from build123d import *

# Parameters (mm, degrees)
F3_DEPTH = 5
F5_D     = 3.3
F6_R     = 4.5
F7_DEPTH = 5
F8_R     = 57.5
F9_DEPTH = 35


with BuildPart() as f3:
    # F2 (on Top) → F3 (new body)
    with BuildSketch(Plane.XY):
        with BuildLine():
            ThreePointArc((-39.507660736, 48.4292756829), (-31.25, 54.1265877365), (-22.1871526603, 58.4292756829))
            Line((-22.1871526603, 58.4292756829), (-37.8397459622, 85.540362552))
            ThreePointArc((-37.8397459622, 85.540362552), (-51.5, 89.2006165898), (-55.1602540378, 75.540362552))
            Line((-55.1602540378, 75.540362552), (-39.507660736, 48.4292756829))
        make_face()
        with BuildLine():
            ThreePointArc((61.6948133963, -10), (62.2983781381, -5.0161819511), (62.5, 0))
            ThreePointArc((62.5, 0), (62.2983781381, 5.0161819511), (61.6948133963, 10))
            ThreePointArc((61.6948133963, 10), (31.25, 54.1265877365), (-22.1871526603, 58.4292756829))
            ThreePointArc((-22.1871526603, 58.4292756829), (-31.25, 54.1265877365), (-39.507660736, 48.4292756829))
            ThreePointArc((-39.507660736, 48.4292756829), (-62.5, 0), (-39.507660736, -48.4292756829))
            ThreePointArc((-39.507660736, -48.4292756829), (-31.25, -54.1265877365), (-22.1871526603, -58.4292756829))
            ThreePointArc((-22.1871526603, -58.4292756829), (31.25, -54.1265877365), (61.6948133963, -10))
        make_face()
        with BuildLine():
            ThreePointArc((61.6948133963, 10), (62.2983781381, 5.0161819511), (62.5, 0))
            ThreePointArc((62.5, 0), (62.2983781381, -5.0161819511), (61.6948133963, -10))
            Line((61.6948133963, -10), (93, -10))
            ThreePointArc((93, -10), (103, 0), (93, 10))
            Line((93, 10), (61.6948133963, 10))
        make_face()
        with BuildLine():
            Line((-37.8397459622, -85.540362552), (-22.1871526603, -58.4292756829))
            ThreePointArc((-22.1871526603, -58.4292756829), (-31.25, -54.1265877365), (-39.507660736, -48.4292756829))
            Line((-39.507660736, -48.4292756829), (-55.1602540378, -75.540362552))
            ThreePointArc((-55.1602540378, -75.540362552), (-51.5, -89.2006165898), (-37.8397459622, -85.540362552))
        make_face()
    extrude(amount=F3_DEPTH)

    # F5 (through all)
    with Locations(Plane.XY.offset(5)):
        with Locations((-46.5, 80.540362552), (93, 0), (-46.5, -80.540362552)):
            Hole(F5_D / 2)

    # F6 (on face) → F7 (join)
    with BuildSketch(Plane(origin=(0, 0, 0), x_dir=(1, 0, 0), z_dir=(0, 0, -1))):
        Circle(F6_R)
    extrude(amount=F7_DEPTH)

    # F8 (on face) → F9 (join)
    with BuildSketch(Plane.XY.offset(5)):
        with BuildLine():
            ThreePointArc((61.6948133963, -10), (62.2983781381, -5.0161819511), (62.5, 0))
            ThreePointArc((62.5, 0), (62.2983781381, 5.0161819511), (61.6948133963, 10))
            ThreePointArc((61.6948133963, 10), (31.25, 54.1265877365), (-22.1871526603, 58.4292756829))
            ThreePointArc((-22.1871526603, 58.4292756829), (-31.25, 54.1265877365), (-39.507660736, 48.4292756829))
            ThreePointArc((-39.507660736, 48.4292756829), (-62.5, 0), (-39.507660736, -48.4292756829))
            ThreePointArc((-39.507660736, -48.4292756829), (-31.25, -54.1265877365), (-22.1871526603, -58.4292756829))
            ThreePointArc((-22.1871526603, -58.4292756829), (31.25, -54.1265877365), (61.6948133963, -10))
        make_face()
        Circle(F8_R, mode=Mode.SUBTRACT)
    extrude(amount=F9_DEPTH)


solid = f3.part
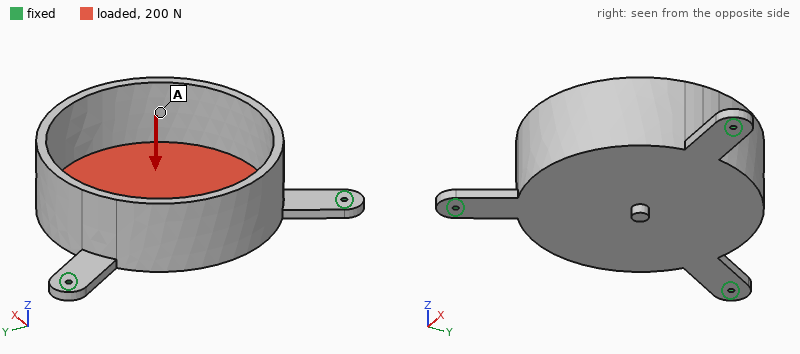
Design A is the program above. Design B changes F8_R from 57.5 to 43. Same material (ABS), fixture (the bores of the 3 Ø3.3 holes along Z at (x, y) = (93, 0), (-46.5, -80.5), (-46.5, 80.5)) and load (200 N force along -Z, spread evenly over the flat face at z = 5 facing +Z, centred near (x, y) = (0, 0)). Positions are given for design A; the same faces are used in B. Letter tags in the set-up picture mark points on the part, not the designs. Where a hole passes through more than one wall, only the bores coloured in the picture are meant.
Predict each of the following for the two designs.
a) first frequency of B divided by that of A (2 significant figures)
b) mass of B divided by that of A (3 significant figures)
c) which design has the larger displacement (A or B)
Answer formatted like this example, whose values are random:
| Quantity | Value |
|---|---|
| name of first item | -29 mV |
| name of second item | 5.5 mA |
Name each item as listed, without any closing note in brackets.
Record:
| Quantity | Value |
|---|---|
| first frequency of B divided by that of A | 0.76 |
| mass of B divided by that of A | 2.15 |
| which design has the larger displacement | A |
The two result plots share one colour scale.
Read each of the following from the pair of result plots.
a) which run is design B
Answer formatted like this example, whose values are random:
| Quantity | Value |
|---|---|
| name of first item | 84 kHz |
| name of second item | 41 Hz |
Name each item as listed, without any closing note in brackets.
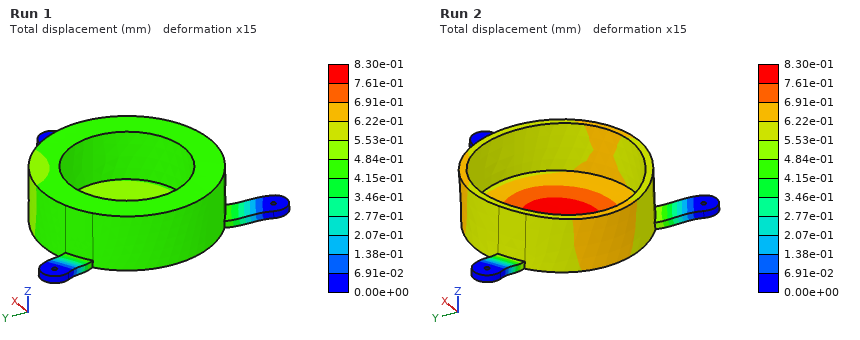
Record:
| Quantity | Value |
|---|---|
| which run is design B | Run 1 |
